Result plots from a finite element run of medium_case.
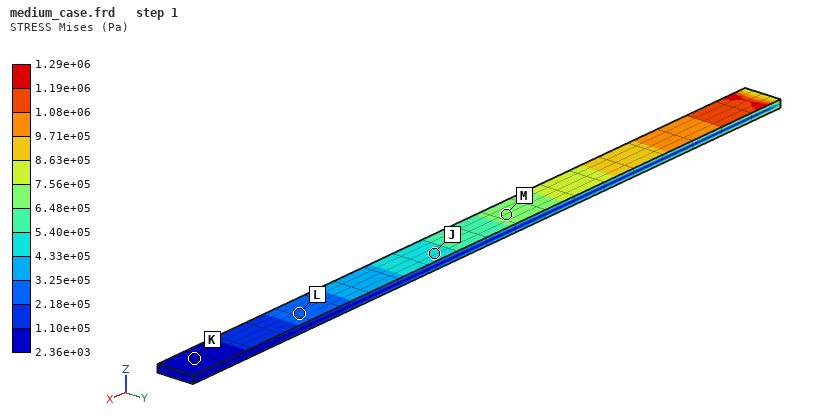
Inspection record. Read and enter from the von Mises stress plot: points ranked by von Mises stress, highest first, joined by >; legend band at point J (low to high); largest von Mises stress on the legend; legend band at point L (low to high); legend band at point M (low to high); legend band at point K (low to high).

M > J > L > K
4.33e+05 to 5.40e+05 Pa
1.29e+06 Pa
2.18e+05 to 3.25e+05 Pa
6.48e+05 to 7.56e+05 Pa
2.36e+03 to 1.10e+05 Pa
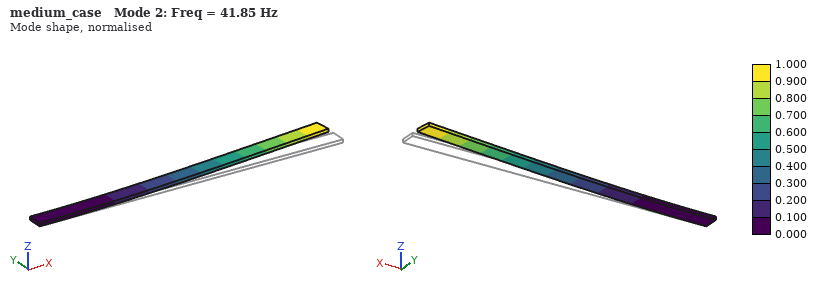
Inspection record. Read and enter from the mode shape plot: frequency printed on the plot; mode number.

41.85 Hz
2
